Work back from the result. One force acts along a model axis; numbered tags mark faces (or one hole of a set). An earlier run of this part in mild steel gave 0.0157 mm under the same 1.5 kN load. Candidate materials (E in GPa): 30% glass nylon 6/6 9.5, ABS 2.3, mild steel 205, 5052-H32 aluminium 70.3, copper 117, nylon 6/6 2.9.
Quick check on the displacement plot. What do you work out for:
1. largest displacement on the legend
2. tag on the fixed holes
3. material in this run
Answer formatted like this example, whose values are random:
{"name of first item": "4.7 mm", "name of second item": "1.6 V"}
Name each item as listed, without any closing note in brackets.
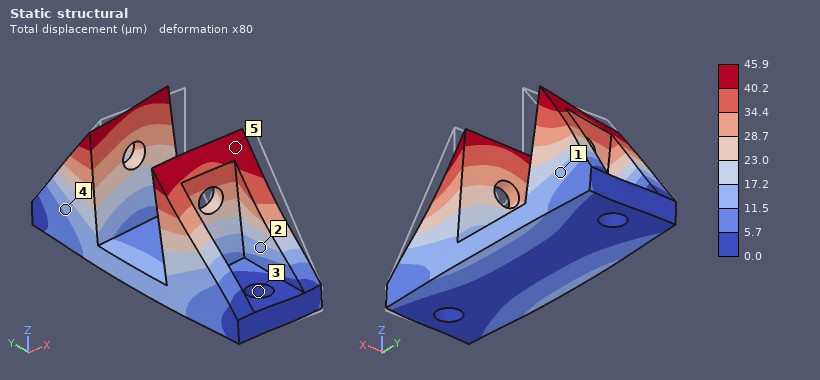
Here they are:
{"largest displacement on the legend": "45.9 µm", "tag on the fixed holes": "3", "material in this run": "5052-H32 aluminium"}
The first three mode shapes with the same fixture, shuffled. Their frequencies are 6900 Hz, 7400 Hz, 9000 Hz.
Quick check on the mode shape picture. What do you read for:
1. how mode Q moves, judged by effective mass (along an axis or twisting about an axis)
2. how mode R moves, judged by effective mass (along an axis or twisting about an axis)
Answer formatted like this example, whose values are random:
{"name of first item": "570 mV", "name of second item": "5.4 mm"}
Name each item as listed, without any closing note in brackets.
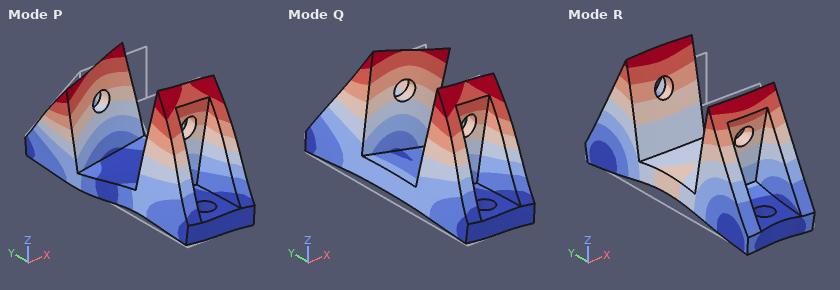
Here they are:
{"how mode Q moves, judged by effective mass": "along X", "how mode R moves, judged by effective mass": "along Z"}
